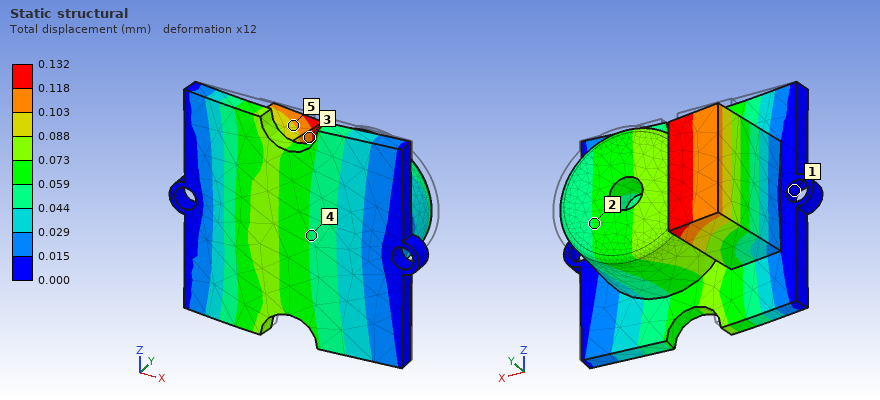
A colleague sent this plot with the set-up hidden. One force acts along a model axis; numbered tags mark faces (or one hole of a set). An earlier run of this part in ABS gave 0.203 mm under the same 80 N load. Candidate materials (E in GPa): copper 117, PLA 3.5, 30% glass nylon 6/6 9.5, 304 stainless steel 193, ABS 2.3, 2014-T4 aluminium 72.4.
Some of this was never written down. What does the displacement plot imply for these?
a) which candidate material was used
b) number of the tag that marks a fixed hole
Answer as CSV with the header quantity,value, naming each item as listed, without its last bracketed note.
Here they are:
quantity,value
which candidate material was used,PLA
number of the tag that marks a fixed hole,1
